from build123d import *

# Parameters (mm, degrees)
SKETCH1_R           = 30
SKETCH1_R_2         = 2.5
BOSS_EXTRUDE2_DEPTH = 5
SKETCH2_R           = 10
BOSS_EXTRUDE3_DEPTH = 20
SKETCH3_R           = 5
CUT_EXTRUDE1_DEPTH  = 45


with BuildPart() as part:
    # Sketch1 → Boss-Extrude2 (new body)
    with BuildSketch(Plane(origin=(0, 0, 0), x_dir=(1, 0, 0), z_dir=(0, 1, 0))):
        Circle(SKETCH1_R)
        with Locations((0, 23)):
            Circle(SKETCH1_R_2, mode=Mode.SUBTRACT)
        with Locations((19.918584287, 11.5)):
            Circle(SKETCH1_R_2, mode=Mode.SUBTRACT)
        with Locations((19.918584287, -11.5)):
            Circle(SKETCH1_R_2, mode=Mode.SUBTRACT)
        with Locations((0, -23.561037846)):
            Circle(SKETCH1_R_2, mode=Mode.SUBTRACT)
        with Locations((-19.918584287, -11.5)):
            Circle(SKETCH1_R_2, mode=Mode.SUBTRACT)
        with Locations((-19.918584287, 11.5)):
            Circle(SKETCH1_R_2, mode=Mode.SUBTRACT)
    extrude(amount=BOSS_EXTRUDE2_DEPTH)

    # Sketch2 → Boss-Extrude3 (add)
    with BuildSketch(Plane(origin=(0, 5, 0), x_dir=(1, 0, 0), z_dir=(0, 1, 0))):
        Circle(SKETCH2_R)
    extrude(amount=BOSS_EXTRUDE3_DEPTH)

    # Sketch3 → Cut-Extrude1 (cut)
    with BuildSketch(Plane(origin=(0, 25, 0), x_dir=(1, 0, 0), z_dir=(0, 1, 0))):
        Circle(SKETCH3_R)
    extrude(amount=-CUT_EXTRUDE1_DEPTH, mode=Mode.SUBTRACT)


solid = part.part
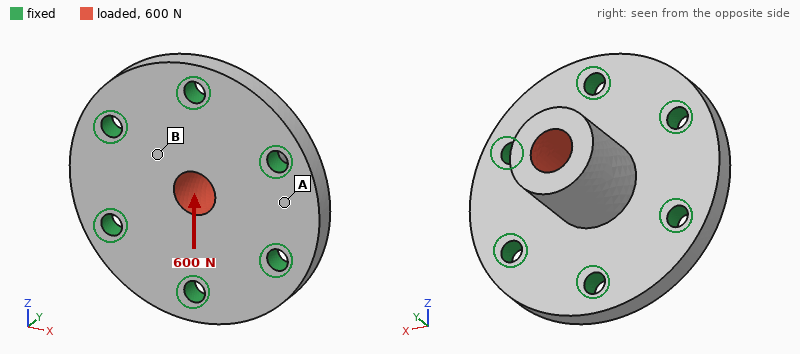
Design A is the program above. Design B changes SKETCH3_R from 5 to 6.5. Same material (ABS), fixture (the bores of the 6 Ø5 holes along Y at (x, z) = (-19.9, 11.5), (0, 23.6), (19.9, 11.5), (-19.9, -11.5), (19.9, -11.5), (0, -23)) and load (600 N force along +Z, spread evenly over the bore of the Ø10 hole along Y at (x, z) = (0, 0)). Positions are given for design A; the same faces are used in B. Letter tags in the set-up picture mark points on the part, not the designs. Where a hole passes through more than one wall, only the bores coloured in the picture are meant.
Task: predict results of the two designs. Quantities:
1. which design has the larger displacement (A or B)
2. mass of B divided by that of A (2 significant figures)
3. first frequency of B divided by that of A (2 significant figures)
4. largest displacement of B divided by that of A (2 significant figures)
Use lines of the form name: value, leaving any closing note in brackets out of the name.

which design has the larger displacement: B
mass of B divided by that of A: 0.92
first frequency of B divided by that of A: 1.0
largest displacement of B divided by that of A: 1.2
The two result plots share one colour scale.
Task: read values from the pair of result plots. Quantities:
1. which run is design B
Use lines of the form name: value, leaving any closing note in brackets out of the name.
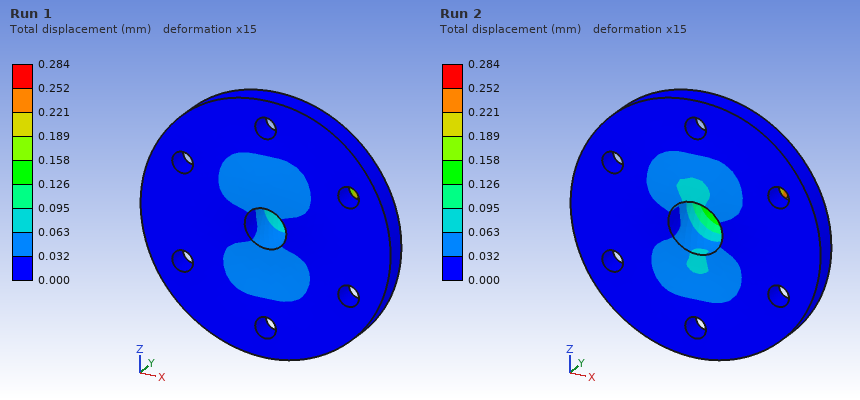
which run is design B: Run 2
